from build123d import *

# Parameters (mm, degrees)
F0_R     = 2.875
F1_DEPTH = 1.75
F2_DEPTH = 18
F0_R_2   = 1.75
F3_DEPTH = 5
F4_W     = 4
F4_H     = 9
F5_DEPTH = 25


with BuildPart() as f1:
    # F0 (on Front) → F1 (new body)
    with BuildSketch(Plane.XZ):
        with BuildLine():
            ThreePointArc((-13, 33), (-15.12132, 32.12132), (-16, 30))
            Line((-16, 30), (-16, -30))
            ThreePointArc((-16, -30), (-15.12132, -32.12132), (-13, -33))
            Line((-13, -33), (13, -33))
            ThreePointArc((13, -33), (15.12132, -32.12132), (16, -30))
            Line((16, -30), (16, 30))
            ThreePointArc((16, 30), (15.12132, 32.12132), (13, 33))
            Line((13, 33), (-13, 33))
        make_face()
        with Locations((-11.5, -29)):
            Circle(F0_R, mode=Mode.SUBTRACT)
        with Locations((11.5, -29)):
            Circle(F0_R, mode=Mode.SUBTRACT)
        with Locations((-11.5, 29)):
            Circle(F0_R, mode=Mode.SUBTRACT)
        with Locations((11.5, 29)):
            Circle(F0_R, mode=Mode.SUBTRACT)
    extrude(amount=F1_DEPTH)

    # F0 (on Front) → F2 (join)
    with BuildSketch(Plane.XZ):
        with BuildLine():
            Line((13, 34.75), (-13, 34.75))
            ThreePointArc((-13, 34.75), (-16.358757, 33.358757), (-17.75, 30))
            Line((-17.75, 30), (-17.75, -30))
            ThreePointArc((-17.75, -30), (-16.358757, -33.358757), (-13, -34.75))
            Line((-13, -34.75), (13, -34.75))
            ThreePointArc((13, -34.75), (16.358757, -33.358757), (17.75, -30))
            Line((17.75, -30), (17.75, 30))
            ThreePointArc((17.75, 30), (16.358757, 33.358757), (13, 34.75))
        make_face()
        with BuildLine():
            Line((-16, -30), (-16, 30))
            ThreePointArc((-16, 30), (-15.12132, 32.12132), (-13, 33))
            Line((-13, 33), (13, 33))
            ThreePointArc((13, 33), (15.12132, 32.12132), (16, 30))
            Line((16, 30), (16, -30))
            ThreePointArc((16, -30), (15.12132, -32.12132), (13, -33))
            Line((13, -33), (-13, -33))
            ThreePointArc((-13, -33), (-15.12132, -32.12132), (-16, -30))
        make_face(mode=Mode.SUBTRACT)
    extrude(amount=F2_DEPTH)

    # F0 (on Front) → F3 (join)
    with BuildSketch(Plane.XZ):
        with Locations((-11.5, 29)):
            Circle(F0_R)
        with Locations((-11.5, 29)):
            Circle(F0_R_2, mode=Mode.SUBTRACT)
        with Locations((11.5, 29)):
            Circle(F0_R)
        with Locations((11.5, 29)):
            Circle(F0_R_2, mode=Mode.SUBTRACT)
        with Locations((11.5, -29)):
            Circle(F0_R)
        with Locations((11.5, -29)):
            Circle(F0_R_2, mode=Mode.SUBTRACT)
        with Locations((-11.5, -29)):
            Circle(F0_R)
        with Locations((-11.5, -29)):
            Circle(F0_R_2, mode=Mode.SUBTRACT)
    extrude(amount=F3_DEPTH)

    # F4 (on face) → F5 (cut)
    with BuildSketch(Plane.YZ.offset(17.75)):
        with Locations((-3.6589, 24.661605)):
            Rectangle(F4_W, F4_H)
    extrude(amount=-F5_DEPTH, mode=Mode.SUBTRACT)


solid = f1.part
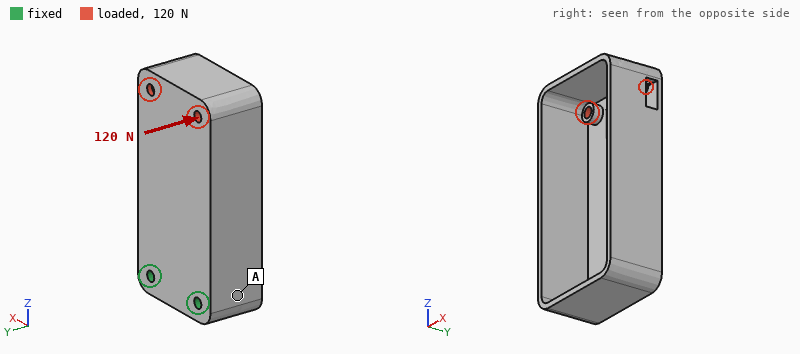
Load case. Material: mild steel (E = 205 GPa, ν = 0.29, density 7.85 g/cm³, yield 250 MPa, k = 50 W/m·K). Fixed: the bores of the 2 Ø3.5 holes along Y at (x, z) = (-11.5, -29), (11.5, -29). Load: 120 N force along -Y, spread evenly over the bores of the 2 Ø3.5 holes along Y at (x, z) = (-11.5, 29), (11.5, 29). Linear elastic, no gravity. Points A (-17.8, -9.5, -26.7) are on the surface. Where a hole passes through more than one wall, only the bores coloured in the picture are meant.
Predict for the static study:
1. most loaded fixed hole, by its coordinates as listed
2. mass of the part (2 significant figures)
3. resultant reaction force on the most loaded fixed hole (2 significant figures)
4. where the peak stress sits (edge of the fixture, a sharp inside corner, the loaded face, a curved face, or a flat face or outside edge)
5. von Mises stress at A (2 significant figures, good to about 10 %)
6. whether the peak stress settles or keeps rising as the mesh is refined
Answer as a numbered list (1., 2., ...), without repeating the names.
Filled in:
1. (-11.5, -29)
2. 78 g
3. 91 N
4. edge of the fixture
5. 18 MPa
6. keeps rising
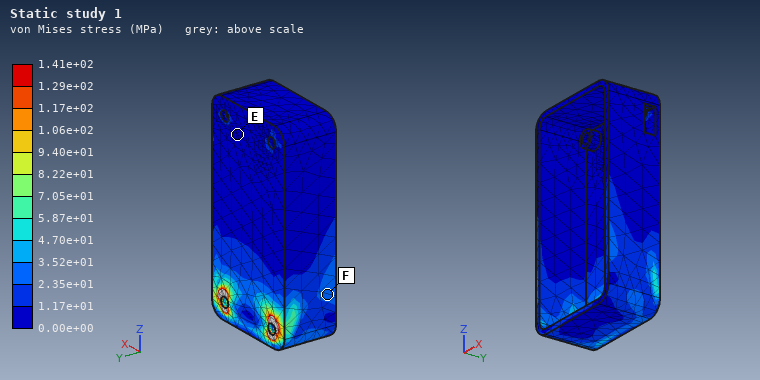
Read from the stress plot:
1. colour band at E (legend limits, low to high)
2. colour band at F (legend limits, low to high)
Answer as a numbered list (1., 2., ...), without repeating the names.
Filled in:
1. 0.00e+00 to 1.17e+01 MPa
2. 2.35e+01 to 3.52e+01 MPa
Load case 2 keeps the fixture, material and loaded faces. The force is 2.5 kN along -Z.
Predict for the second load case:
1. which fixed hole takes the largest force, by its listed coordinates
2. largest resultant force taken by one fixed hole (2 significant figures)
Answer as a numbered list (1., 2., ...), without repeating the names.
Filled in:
1. (-11.5, -29)
2. 1.5 kN
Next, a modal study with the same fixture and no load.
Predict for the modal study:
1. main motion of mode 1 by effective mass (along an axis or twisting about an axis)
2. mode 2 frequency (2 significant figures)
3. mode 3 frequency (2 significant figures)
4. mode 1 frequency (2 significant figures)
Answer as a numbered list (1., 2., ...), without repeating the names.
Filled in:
1. along Y
2. 1300 Hz
3. 3800 Hz
4. 800 Hz
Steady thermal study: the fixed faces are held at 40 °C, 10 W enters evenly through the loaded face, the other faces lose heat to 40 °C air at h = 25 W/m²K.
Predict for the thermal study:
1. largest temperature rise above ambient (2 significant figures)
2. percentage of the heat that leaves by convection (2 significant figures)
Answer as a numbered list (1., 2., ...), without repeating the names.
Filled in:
1. 73 K
2. 69 %
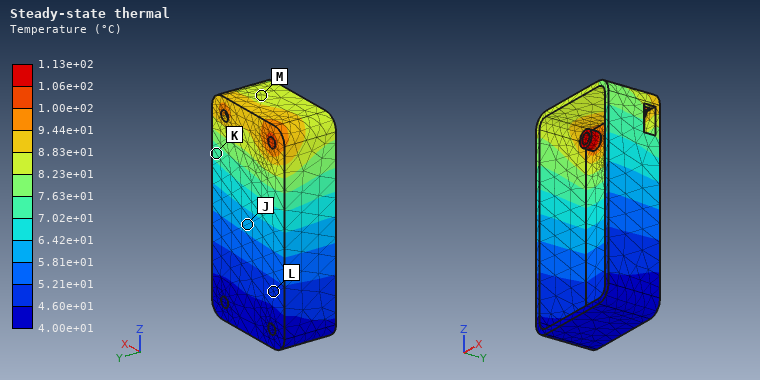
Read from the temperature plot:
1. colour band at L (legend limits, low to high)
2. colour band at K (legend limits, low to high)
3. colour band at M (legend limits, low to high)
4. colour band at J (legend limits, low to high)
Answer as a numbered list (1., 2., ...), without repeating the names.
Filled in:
1. 4.60e+01 to 5.21e+01 °C
2. 7.02e+01 to 7.63e+01 °C
3. 8.23e+01 to 8.83e+01 °C
4. 5.81e+01 to 6.42e+01 °C
